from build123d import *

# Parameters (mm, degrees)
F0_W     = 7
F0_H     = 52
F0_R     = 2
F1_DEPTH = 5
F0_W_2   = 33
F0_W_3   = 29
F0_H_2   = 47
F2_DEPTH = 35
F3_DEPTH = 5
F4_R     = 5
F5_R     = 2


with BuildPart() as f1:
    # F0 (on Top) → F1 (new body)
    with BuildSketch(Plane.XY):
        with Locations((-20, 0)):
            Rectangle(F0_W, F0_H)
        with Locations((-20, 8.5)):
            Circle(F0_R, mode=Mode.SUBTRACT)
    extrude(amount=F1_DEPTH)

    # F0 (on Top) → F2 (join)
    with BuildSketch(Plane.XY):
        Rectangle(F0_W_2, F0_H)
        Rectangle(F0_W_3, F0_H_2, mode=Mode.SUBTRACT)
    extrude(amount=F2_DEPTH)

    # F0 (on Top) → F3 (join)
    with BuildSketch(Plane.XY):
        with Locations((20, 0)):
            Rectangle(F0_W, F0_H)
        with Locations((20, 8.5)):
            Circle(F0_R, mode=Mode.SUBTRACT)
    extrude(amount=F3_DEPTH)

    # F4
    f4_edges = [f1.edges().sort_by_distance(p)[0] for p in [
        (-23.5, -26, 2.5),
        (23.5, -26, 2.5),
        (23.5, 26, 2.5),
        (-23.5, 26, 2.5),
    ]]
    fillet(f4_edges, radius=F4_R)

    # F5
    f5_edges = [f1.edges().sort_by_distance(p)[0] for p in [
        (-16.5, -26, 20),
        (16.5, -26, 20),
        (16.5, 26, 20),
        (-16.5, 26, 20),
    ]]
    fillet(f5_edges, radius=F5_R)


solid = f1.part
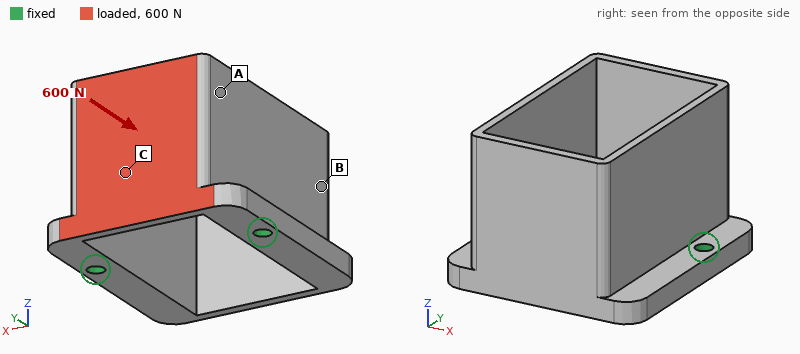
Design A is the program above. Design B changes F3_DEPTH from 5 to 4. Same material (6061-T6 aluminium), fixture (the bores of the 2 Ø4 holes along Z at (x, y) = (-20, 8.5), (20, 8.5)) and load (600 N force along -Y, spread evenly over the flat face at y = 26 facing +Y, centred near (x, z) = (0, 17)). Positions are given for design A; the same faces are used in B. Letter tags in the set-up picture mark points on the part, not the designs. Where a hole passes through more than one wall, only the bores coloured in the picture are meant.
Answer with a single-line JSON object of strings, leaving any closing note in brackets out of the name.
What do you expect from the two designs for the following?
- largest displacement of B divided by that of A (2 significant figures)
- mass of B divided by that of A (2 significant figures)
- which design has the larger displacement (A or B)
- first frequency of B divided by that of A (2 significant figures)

{"largest displacement of B divided by that of A": "1.1", "mass of B divided by that of A": "0.98", "which design has the larger displacement": "B", "first frequency of B divided by that of A": "0.88"}
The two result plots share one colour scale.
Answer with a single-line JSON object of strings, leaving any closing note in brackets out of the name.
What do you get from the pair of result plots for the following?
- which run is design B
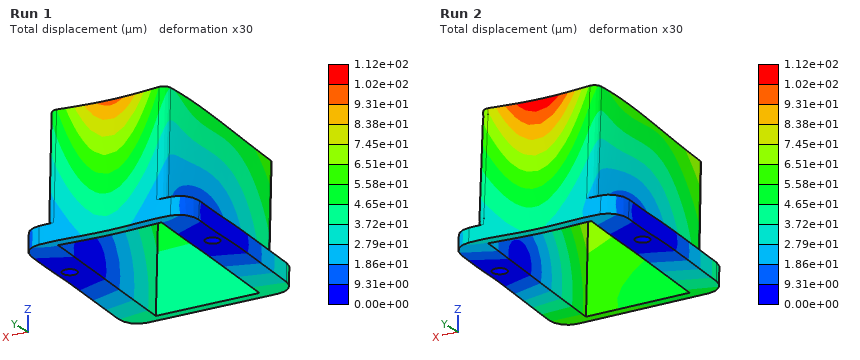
{"which run is design B": "Run 2"}
